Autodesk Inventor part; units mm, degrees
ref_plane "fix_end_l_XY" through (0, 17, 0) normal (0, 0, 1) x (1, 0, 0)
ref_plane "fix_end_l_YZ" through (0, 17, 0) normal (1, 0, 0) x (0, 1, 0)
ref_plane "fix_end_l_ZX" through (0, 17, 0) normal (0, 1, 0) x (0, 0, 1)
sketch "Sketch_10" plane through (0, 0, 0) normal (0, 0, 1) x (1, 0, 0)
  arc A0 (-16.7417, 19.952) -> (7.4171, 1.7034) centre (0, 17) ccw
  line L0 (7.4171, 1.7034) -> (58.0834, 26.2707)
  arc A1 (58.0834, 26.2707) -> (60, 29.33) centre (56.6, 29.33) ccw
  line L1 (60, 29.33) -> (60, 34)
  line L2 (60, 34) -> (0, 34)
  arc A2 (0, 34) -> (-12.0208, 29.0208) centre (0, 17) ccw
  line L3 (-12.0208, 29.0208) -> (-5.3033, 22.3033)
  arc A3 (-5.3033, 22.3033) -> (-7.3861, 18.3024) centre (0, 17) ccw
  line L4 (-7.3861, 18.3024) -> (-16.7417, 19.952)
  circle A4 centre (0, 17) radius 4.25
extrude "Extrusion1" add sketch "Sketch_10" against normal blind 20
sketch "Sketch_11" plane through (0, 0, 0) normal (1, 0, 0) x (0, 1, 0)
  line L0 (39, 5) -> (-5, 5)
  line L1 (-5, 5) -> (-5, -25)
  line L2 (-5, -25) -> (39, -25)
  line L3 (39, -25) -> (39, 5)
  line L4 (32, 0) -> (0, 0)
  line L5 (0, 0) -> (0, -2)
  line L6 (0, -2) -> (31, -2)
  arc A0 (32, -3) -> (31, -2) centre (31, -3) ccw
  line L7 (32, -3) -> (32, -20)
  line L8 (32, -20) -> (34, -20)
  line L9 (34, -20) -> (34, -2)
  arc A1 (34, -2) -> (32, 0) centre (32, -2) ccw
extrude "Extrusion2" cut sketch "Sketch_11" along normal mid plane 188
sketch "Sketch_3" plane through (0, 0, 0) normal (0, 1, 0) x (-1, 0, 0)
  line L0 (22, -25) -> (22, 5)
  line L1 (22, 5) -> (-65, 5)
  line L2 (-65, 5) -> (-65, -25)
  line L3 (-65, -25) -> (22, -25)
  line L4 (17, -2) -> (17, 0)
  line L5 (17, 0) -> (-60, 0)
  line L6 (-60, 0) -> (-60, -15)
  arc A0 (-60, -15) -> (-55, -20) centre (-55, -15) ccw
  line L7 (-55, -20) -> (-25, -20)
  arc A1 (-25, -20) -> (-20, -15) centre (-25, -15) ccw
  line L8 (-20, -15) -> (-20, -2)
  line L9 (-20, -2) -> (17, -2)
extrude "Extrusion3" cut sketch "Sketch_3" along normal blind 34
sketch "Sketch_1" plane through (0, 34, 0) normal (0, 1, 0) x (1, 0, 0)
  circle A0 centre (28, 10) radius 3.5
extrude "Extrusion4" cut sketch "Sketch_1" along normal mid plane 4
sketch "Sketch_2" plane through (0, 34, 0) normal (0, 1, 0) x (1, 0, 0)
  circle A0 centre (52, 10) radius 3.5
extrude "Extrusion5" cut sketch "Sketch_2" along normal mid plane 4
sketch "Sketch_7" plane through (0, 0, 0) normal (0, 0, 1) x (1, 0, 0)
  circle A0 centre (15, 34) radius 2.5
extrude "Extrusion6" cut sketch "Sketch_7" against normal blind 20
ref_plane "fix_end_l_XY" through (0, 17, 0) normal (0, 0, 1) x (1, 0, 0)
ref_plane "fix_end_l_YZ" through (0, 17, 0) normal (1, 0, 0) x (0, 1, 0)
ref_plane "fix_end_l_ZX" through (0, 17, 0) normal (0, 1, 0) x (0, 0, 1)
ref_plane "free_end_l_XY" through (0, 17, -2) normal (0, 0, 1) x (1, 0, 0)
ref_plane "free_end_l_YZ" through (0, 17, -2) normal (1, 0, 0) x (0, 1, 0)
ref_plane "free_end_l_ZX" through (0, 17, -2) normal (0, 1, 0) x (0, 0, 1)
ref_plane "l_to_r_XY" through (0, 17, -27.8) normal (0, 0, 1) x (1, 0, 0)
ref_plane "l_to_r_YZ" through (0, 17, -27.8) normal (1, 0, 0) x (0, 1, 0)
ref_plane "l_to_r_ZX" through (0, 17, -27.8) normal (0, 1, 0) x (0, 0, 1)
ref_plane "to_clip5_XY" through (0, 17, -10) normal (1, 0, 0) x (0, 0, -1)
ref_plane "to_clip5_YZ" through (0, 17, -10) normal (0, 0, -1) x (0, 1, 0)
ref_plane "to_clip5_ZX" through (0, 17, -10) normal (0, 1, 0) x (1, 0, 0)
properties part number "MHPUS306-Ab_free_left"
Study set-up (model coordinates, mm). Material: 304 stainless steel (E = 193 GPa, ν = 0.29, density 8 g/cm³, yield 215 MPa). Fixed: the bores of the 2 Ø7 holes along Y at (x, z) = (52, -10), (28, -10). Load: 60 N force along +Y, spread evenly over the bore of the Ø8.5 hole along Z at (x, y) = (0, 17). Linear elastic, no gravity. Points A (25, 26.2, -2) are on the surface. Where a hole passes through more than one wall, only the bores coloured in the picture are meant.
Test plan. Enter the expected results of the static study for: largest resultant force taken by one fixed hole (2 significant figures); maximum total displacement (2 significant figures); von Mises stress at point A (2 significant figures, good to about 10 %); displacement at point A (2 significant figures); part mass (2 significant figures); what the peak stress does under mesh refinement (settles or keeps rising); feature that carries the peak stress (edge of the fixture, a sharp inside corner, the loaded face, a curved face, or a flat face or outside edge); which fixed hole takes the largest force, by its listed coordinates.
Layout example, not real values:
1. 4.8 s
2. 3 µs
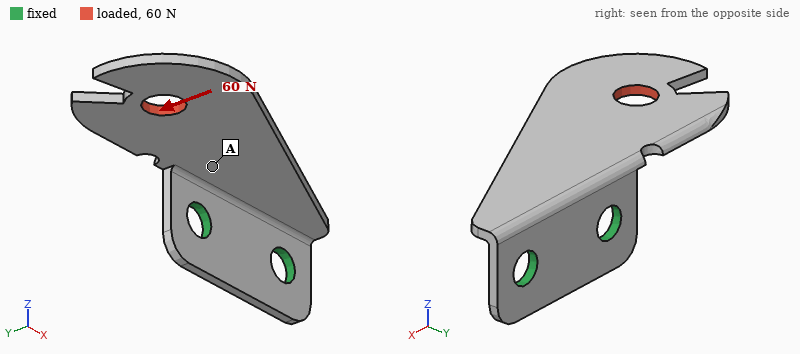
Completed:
1. 120 N
2. 37 µm
3. 7.1 MPa
4. 7.0 µm
5. 35 g
6. keeps rising
7. edge of the fixture
8. (28, -10)
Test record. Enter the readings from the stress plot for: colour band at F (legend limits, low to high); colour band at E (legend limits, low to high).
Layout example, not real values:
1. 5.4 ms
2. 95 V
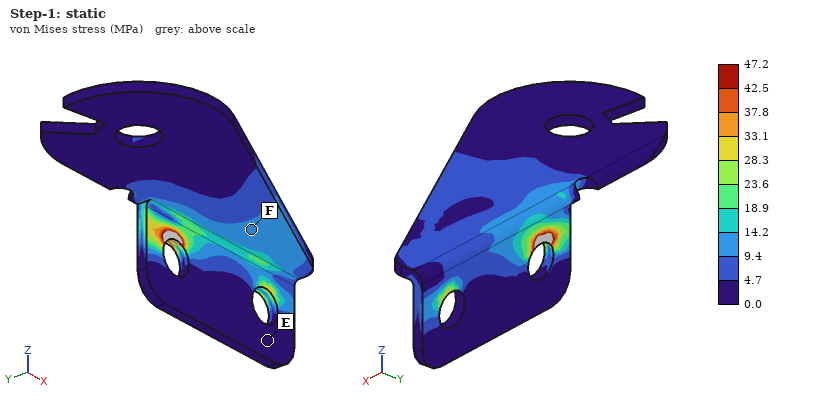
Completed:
1. 9.4 to 14.2 MPa
2. 0.0 to 4.7 MPa
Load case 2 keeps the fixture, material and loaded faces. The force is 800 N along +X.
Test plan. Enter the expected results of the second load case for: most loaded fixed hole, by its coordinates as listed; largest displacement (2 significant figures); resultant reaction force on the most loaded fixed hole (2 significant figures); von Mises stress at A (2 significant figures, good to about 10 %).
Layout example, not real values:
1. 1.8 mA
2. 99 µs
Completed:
1. (52, -10)
2. 0.15 mm
3. 700 N
4. 42 MPa
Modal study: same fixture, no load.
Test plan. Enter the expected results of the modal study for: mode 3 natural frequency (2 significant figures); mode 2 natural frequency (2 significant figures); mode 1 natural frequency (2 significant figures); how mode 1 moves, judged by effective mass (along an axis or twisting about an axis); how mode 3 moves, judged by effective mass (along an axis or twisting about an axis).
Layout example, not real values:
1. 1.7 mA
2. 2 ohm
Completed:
1. 2700 Hz
2. 1900 Hz
3. 670 Hz
4. along Z
5. along Y
